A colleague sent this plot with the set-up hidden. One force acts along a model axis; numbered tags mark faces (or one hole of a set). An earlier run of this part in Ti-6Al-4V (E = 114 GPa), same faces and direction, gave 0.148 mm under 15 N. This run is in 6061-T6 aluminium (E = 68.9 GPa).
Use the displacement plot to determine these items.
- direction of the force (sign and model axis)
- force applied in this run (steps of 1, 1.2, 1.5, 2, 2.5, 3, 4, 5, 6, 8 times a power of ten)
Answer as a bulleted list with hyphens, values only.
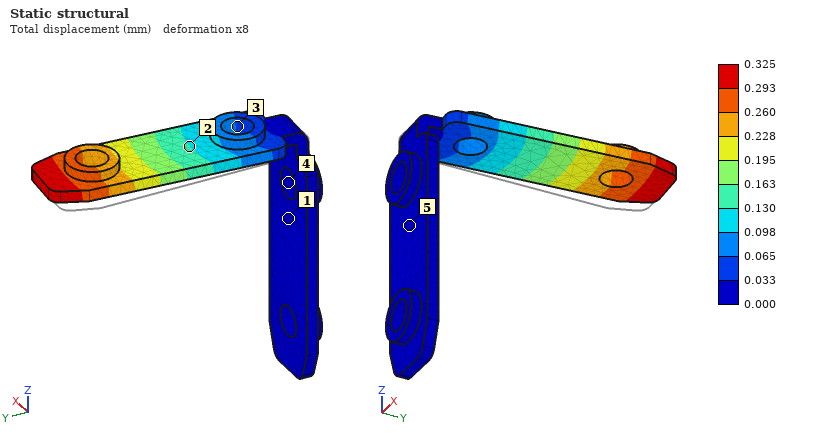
- +X
- 20 N
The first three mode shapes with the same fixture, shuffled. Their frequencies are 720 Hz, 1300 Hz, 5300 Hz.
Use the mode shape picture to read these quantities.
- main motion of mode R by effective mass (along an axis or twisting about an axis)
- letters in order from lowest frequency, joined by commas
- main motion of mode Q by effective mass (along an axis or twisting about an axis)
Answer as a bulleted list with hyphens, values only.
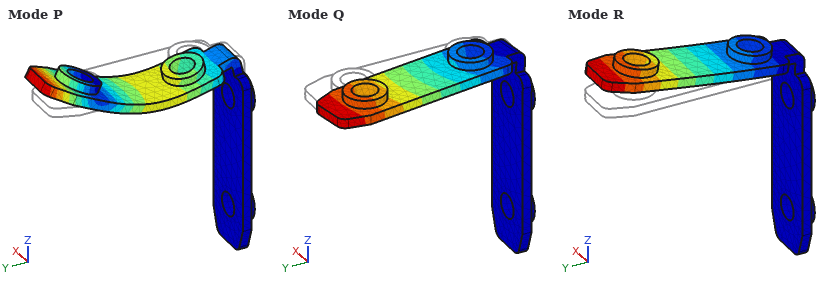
- along Z
- R, Q, P
- along X
